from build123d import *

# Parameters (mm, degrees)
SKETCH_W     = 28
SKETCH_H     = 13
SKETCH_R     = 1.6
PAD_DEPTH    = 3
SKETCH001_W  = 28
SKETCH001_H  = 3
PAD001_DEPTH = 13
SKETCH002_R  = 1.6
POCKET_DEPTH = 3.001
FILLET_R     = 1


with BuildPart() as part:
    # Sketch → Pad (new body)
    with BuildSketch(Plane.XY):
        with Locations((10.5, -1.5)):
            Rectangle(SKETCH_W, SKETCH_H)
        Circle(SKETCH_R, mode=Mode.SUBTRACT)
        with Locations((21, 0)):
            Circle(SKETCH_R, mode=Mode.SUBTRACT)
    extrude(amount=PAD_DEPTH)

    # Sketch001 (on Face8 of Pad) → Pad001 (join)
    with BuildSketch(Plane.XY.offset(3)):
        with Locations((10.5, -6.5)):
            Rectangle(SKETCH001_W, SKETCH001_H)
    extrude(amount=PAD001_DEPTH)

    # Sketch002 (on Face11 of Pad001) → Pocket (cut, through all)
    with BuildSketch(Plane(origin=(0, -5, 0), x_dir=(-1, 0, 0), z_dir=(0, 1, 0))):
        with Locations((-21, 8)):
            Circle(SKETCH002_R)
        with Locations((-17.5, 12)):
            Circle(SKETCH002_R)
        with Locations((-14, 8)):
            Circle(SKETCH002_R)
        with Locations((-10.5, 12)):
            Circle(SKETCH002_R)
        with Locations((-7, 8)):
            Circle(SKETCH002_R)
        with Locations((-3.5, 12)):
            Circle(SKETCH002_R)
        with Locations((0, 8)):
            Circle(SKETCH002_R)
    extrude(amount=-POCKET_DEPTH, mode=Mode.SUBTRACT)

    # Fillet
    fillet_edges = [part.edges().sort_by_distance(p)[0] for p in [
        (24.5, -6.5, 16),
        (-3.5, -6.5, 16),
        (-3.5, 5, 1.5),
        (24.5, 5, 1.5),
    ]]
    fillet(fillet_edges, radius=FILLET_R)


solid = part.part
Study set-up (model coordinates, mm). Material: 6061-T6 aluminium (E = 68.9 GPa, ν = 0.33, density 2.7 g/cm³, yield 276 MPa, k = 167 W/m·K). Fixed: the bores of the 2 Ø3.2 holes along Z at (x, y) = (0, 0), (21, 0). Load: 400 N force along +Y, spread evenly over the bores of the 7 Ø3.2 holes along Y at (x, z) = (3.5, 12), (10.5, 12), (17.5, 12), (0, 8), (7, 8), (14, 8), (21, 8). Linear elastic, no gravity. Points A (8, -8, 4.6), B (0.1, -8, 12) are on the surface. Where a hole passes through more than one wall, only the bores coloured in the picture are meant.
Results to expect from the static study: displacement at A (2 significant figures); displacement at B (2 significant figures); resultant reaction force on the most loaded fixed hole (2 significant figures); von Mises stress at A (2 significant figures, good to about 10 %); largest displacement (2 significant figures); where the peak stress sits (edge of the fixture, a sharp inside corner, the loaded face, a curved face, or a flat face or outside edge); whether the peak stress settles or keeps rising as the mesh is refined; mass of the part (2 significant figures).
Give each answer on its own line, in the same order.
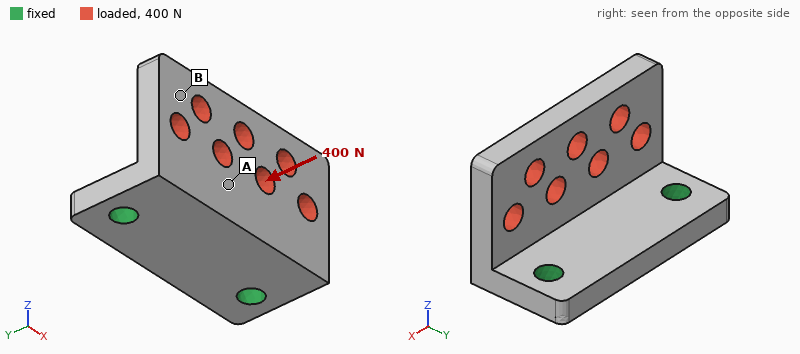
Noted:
0.031 mm
0.075 mm
210 N
44 MPa
0.11 mm
edge of the fixture
keeps rising
5.3 g
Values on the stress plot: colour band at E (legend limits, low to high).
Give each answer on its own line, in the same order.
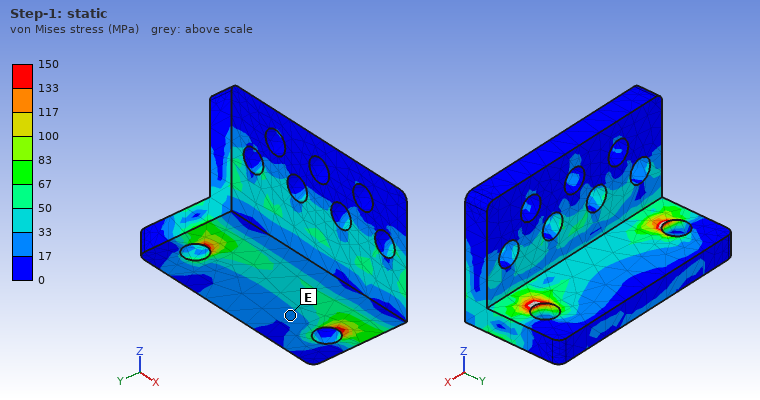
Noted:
17 to 33 MPa
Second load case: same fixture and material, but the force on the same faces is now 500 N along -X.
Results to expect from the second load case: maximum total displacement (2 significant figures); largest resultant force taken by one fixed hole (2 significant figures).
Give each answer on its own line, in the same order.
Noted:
20 µm
340 N
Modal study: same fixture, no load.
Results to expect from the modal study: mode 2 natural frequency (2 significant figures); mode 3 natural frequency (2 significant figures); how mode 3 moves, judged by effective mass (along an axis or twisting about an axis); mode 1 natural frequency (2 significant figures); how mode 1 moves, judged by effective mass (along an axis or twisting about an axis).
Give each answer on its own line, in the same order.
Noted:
13 kHz
21 kHz
along X
7200 Hz
along Y
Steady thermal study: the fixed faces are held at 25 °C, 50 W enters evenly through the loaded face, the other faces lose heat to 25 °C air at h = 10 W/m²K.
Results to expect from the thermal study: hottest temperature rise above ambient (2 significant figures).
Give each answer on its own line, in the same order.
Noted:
65 K
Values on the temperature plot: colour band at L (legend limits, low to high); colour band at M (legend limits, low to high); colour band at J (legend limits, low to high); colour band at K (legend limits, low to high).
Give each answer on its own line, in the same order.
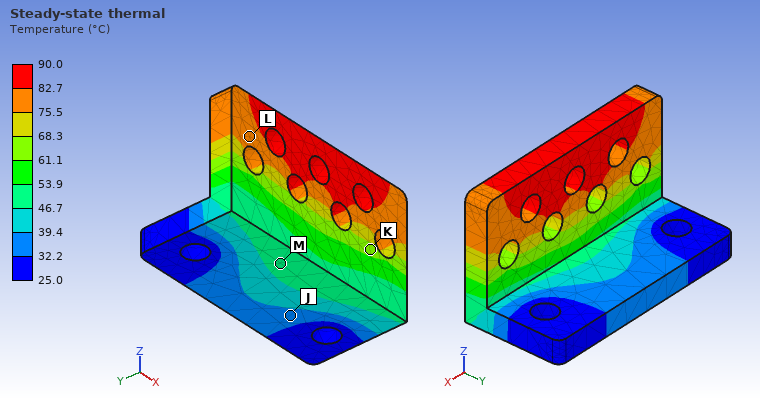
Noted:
75.5 to 82.7 °C
46.7 to 53.9 °C
32.2 to 39.4 °C
61.1 to 68.3 °C
